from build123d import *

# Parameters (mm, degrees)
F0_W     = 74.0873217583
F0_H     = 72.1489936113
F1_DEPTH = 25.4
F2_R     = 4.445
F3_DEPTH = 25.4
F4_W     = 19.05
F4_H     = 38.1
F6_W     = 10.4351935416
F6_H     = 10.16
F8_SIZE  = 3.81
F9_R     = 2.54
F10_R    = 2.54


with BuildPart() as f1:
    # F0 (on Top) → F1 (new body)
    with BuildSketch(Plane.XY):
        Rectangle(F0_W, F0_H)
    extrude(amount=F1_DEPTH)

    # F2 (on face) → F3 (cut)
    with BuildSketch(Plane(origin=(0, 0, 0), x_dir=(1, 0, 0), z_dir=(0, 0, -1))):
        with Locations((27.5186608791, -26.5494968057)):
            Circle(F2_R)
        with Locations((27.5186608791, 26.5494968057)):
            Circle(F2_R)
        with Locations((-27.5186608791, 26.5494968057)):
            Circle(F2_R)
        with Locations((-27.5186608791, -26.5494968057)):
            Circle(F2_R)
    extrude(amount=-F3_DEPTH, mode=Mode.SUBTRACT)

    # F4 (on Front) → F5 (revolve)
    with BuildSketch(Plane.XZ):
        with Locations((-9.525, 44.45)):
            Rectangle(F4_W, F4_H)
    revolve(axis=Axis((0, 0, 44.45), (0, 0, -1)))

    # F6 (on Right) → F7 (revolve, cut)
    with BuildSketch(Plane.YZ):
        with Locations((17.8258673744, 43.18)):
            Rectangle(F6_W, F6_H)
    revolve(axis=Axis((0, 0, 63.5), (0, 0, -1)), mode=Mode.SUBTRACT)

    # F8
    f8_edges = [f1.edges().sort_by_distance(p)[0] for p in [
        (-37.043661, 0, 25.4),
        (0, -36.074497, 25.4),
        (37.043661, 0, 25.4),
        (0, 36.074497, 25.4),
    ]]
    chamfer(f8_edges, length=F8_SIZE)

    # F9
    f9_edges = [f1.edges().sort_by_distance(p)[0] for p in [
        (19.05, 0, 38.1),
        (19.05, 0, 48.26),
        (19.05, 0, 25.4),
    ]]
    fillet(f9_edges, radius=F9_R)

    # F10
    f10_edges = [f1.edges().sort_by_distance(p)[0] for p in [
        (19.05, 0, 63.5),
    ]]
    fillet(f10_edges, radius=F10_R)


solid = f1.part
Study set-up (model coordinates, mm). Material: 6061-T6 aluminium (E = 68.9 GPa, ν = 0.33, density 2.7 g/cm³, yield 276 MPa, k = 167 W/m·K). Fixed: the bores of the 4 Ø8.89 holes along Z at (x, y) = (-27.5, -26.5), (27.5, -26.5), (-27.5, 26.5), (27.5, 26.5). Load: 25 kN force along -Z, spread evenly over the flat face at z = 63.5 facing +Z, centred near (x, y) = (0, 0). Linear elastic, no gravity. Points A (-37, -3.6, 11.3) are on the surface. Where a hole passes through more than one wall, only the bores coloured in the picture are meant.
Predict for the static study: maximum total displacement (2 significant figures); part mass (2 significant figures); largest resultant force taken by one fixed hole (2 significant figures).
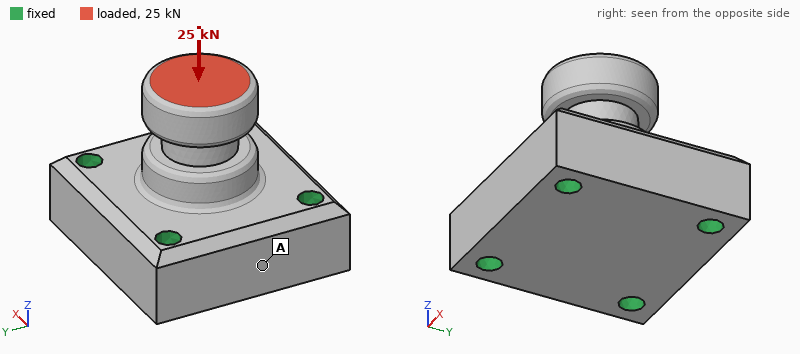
32 µm
440 g
6.5 kN
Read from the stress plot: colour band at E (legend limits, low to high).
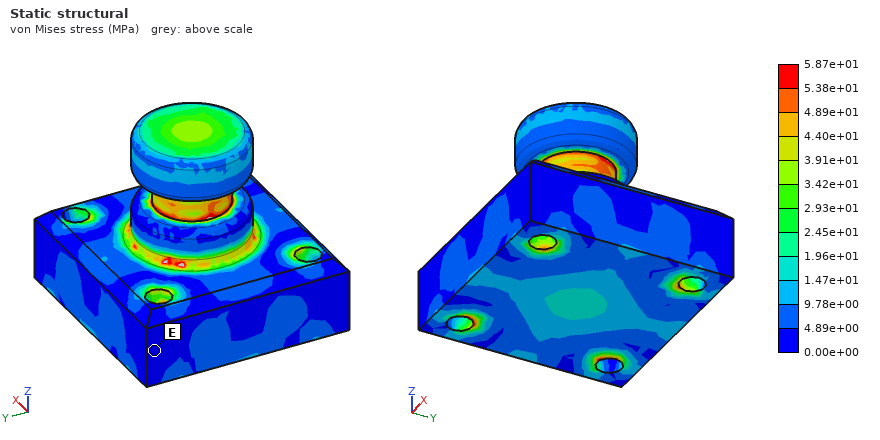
0.00e+00 to 4.89e+00 MPa
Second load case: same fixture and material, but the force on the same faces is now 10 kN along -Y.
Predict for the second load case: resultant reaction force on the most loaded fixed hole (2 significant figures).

5.6 kN
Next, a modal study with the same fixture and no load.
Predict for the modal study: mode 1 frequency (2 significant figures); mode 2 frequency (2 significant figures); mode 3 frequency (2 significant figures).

8000 Hz
8000 Hz
13 kHz
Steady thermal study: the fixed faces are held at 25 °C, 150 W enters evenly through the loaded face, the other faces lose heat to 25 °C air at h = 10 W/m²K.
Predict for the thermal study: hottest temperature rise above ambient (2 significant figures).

59 K
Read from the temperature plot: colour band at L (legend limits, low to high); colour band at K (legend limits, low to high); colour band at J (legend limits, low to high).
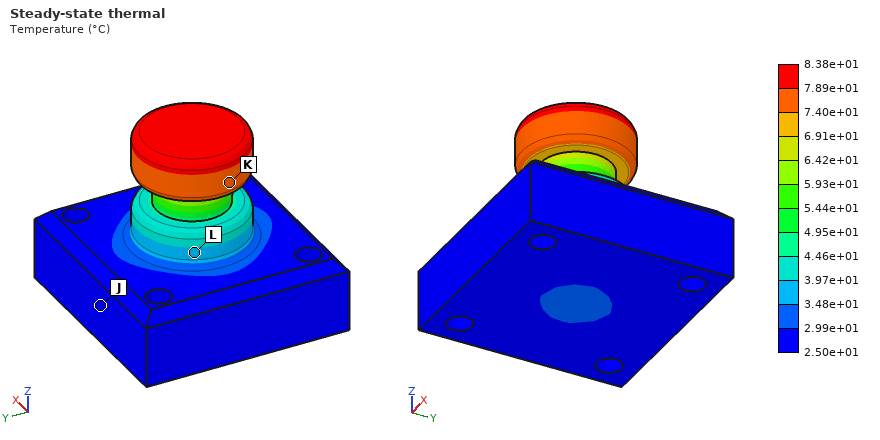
3.48e+01 to 3.97e+01 °C
7.40e+01 to 7.89e+01 °C
2.50e+01 to 2.99e+01 °C
